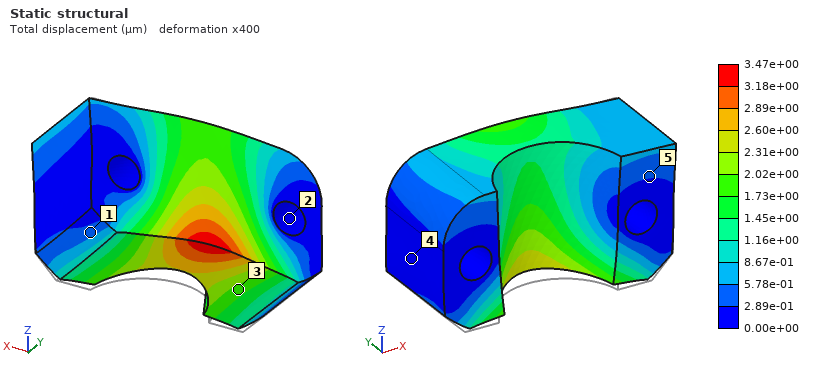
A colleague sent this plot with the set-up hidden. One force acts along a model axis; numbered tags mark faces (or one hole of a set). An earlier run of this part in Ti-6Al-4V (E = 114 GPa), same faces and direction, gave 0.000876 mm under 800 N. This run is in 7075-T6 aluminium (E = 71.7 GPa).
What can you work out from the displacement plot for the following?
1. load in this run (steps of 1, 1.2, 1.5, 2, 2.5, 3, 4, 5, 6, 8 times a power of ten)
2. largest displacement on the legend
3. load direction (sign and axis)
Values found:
2 kN
3.47e+00 µm
+Z
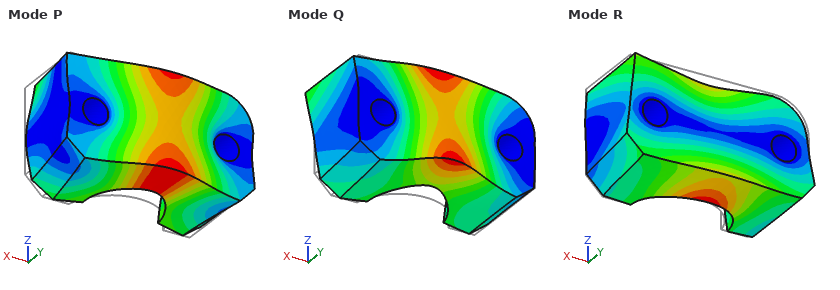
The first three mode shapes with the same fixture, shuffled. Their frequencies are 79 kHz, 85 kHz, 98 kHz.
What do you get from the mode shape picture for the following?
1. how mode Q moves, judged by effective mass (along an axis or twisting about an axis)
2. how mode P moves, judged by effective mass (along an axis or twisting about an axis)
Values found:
along Z
along Y
